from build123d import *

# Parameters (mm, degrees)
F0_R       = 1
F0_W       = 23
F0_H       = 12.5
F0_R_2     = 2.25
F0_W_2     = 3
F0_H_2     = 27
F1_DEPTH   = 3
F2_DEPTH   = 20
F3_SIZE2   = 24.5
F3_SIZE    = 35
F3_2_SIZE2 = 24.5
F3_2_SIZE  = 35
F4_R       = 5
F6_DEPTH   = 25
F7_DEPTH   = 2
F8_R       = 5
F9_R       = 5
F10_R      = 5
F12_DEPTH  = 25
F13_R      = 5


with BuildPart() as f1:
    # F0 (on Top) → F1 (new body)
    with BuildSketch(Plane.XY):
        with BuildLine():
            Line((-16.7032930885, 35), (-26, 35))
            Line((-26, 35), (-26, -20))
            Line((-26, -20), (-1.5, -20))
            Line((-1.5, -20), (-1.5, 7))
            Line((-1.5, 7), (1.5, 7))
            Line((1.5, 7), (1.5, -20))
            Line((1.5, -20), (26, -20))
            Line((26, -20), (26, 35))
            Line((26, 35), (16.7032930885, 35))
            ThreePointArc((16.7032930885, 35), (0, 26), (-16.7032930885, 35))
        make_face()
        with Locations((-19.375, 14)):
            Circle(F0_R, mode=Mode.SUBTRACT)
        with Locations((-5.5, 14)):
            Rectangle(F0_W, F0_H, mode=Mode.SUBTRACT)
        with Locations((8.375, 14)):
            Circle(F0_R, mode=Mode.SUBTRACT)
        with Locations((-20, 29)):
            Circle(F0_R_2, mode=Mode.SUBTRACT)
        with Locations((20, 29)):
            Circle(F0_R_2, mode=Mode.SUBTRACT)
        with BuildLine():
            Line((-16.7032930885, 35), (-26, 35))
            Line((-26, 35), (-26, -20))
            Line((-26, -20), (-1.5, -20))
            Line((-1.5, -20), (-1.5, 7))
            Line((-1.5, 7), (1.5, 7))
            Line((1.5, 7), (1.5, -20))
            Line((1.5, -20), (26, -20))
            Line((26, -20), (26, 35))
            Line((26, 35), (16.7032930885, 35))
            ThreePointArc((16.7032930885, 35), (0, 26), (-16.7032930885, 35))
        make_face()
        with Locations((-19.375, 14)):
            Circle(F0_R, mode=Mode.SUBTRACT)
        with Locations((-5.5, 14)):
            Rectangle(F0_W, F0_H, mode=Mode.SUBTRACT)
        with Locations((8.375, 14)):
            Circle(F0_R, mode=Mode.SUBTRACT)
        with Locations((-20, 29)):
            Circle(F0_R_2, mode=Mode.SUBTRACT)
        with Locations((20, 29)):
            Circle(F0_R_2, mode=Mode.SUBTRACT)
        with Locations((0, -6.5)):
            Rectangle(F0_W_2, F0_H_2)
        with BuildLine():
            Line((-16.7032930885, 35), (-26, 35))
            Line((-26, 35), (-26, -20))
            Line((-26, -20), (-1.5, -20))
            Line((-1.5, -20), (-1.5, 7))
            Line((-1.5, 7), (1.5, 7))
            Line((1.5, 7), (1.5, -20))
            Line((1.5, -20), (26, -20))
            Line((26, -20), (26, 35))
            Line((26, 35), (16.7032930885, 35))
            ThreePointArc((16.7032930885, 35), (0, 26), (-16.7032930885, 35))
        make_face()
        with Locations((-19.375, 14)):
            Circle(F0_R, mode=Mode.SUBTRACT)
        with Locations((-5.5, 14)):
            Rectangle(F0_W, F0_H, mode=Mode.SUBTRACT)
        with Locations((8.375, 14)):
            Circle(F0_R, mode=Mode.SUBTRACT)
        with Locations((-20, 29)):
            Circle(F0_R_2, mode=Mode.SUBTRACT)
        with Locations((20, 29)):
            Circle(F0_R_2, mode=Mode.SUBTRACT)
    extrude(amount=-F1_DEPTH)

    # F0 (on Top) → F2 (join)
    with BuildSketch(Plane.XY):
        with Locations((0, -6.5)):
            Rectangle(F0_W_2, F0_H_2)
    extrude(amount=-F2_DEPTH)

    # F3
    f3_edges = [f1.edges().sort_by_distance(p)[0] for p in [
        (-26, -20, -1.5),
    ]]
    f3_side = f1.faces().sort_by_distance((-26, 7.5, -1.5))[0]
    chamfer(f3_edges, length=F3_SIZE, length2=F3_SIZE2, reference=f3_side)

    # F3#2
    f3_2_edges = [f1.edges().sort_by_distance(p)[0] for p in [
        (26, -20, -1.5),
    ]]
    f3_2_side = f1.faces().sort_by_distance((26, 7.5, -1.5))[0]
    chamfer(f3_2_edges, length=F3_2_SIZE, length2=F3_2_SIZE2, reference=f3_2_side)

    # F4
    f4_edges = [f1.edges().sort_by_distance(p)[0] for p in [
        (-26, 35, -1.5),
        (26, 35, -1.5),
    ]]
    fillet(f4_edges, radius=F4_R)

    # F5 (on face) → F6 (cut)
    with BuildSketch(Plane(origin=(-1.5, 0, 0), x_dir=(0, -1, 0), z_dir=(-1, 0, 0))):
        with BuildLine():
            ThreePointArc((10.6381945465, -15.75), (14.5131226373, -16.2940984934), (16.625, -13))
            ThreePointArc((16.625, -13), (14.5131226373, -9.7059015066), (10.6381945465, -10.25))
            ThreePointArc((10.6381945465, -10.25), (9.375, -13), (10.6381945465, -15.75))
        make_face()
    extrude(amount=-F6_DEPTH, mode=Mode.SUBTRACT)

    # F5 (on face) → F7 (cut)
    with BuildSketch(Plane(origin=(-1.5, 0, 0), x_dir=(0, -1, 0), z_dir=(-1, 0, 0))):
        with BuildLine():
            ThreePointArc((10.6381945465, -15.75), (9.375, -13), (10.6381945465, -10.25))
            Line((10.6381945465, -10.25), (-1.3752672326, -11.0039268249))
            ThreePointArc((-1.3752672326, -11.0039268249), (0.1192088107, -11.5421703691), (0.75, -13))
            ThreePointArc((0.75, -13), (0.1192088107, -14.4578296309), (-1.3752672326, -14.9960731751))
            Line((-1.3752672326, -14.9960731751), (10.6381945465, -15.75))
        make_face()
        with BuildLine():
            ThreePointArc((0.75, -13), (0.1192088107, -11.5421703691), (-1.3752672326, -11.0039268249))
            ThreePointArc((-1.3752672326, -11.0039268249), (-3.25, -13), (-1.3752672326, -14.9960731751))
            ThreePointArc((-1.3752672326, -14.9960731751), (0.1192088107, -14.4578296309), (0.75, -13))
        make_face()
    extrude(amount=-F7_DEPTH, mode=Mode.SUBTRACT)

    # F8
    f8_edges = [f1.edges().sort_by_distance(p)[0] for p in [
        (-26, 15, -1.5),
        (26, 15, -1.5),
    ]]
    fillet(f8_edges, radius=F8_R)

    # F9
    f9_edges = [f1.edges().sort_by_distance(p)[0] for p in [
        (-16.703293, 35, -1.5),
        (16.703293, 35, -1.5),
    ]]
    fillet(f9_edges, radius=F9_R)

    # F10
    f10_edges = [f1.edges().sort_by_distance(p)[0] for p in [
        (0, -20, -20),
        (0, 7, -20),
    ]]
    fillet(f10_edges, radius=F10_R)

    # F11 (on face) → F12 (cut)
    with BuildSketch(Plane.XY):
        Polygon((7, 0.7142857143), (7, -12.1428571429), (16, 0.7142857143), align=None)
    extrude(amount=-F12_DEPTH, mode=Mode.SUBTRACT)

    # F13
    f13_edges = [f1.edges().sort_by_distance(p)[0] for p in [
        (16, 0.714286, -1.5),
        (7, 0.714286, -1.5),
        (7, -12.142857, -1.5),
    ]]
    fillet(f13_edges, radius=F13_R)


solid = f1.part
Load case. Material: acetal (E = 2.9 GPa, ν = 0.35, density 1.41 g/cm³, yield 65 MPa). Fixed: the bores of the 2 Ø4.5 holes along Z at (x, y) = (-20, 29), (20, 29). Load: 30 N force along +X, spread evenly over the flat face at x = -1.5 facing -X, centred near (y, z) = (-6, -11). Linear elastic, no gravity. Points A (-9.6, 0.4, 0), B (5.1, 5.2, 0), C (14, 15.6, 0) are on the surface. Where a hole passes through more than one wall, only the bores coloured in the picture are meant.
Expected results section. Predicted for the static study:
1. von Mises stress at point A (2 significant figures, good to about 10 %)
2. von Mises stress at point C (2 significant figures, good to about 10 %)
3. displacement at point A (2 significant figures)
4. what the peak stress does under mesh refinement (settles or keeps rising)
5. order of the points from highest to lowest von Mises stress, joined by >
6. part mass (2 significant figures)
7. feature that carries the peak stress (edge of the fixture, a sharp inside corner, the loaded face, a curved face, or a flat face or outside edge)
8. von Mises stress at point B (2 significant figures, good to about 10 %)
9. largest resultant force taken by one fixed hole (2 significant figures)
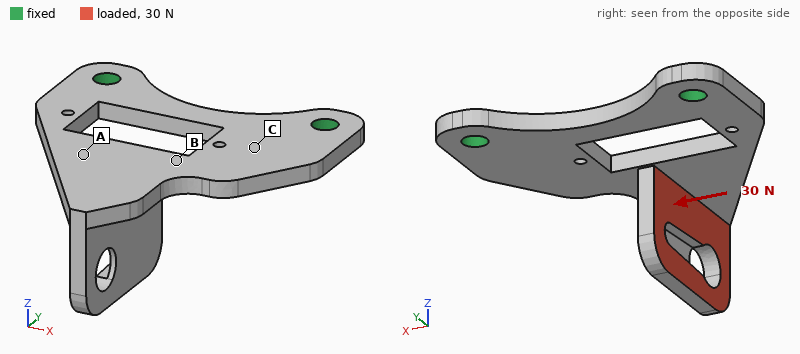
4.5 MPa
1.9 MPa
0.20 mm
keeps rising
B > A > C
7.5 g
a sharp inside corner
6.3 MPa
27 N
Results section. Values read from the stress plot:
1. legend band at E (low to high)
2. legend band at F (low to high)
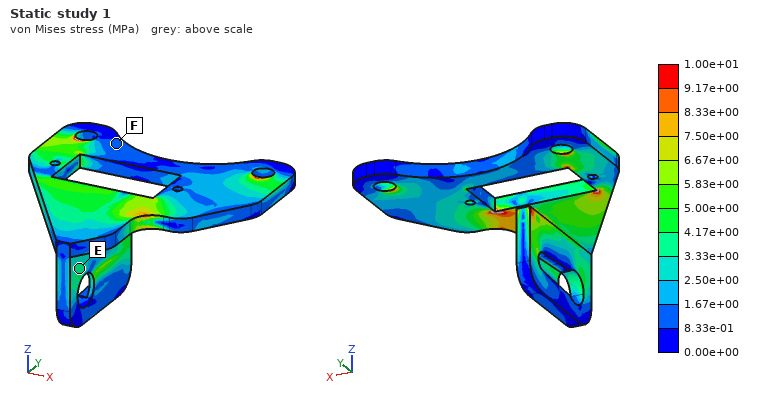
3.33e+00 to 4.17e+00 MPa
8.33e-01 to 1.67e+00 MPa
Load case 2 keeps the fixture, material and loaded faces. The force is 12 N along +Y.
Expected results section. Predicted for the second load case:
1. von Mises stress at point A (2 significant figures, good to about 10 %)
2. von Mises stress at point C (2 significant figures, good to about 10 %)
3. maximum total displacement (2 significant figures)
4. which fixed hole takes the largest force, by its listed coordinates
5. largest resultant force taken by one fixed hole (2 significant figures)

1.2 MPa
2.8 MPa
0.88 mm
(20, 29)
6.8 N
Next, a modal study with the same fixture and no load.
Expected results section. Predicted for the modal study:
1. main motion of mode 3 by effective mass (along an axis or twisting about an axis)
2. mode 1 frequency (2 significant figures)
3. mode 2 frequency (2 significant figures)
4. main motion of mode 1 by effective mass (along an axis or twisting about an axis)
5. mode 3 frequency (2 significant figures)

along Z
260 Hz
920 Hz
along Z
1100 Hz
